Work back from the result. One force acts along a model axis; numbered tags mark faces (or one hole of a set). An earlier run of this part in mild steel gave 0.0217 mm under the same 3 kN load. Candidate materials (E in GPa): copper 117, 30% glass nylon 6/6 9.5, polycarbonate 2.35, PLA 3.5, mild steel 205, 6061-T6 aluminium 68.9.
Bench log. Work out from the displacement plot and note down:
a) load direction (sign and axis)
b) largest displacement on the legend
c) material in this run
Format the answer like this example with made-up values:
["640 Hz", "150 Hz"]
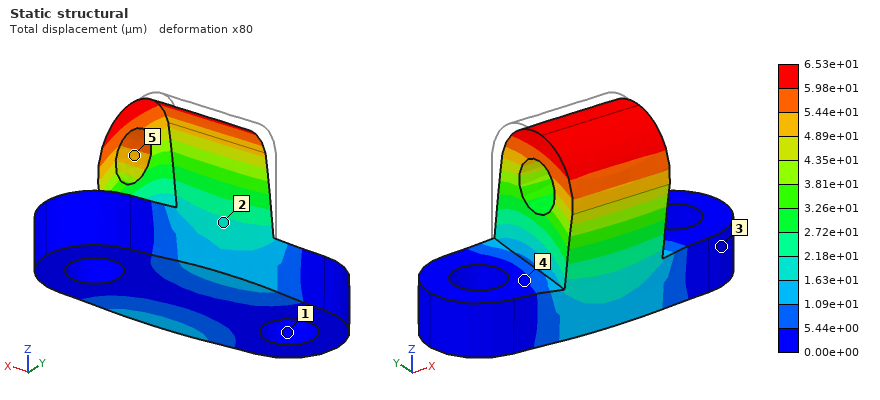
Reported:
["-Y", "6.53e+01 µm", "6061-T6 aluminium"]
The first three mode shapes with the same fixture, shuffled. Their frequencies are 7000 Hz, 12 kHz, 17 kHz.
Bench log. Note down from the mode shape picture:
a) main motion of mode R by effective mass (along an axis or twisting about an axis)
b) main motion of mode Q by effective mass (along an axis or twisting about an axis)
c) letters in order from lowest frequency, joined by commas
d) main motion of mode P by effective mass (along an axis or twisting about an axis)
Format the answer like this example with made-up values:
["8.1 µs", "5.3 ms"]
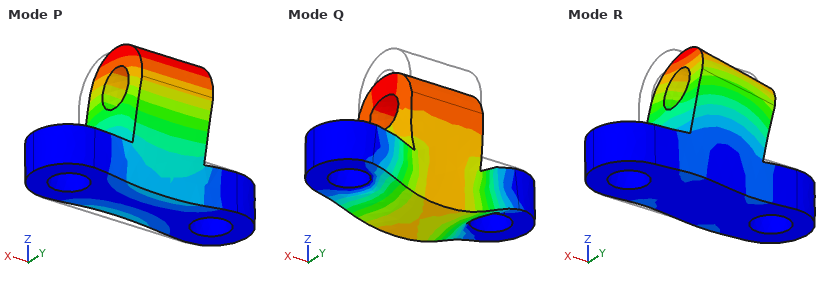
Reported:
["along X", "along Z", "P, R, Q", "along Y"]
